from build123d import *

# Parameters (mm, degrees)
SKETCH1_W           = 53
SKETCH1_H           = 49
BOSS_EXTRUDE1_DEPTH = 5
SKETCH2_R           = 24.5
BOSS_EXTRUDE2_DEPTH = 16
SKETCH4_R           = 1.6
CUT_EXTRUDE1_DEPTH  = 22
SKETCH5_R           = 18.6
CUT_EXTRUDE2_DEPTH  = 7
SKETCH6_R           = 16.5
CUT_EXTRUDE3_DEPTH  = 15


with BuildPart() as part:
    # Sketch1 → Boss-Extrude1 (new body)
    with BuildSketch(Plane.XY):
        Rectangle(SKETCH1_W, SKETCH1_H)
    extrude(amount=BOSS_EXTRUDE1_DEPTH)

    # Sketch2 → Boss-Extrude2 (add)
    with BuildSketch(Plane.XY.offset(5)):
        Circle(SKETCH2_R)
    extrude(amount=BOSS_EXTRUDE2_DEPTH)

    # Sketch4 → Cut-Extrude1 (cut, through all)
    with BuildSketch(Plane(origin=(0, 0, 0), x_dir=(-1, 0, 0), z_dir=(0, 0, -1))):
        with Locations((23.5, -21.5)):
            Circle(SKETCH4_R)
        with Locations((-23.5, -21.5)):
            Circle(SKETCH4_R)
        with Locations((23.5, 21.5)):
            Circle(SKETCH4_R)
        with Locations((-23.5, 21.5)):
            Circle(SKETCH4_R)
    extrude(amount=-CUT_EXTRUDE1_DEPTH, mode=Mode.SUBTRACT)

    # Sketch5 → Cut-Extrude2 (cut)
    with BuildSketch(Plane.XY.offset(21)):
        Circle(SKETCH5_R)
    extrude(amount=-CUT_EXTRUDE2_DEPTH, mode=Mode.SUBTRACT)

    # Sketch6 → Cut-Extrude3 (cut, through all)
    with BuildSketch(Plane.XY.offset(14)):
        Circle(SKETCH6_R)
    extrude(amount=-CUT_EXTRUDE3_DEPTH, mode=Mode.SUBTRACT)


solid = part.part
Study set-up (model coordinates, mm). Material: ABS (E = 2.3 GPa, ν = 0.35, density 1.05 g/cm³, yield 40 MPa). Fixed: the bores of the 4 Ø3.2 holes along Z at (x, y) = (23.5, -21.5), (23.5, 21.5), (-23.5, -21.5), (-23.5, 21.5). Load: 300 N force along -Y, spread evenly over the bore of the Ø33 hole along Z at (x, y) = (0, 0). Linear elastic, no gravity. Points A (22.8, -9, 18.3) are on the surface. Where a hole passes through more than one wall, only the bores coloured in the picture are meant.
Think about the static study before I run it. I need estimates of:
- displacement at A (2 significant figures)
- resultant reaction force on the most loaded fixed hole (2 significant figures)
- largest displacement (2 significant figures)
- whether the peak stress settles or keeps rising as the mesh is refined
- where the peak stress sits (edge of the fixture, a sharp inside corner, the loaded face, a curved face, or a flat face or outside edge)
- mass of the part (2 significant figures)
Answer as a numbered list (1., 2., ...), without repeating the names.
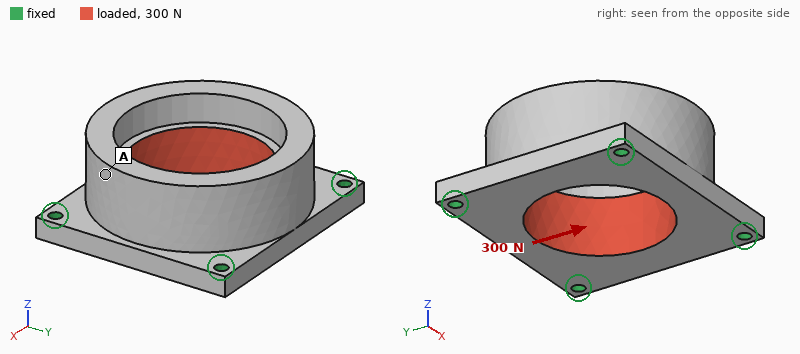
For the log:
1. 17 µm
2. 81 N
3. 23 µm
4. keeps rising
5. edge of the fixture
6. 25 g
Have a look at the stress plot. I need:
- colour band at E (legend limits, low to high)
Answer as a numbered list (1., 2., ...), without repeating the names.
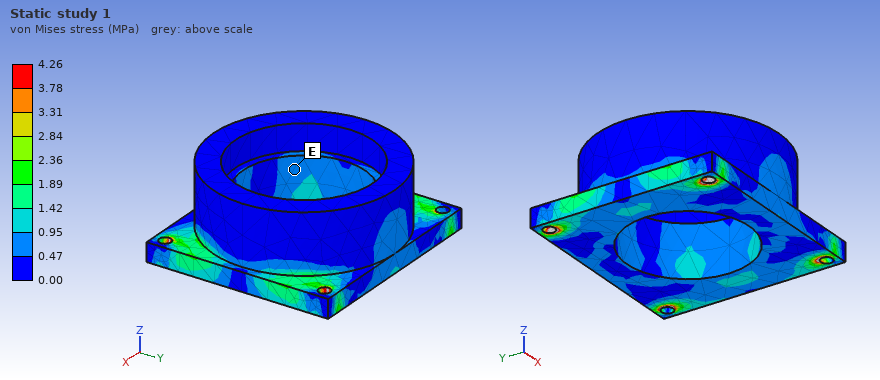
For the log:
1. 0.47 to 0.95 MPa
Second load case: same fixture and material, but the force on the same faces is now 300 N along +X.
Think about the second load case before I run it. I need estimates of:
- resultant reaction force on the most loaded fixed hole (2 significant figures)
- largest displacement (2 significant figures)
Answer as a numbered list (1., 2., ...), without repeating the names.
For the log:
1. 80 N
2. 21 µm
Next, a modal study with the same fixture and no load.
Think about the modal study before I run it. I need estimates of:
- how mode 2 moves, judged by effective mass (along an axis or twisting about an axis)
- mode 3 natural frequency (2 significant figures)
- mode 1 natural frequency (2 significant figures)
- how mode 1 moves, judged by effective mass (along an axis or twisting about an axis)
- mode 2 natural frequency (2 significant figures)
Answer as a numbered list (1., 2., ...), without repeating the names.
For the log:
1. along Y
2. 3400 Hz
3. 3000 Hz
4. along Z
5. 3200 Hz
